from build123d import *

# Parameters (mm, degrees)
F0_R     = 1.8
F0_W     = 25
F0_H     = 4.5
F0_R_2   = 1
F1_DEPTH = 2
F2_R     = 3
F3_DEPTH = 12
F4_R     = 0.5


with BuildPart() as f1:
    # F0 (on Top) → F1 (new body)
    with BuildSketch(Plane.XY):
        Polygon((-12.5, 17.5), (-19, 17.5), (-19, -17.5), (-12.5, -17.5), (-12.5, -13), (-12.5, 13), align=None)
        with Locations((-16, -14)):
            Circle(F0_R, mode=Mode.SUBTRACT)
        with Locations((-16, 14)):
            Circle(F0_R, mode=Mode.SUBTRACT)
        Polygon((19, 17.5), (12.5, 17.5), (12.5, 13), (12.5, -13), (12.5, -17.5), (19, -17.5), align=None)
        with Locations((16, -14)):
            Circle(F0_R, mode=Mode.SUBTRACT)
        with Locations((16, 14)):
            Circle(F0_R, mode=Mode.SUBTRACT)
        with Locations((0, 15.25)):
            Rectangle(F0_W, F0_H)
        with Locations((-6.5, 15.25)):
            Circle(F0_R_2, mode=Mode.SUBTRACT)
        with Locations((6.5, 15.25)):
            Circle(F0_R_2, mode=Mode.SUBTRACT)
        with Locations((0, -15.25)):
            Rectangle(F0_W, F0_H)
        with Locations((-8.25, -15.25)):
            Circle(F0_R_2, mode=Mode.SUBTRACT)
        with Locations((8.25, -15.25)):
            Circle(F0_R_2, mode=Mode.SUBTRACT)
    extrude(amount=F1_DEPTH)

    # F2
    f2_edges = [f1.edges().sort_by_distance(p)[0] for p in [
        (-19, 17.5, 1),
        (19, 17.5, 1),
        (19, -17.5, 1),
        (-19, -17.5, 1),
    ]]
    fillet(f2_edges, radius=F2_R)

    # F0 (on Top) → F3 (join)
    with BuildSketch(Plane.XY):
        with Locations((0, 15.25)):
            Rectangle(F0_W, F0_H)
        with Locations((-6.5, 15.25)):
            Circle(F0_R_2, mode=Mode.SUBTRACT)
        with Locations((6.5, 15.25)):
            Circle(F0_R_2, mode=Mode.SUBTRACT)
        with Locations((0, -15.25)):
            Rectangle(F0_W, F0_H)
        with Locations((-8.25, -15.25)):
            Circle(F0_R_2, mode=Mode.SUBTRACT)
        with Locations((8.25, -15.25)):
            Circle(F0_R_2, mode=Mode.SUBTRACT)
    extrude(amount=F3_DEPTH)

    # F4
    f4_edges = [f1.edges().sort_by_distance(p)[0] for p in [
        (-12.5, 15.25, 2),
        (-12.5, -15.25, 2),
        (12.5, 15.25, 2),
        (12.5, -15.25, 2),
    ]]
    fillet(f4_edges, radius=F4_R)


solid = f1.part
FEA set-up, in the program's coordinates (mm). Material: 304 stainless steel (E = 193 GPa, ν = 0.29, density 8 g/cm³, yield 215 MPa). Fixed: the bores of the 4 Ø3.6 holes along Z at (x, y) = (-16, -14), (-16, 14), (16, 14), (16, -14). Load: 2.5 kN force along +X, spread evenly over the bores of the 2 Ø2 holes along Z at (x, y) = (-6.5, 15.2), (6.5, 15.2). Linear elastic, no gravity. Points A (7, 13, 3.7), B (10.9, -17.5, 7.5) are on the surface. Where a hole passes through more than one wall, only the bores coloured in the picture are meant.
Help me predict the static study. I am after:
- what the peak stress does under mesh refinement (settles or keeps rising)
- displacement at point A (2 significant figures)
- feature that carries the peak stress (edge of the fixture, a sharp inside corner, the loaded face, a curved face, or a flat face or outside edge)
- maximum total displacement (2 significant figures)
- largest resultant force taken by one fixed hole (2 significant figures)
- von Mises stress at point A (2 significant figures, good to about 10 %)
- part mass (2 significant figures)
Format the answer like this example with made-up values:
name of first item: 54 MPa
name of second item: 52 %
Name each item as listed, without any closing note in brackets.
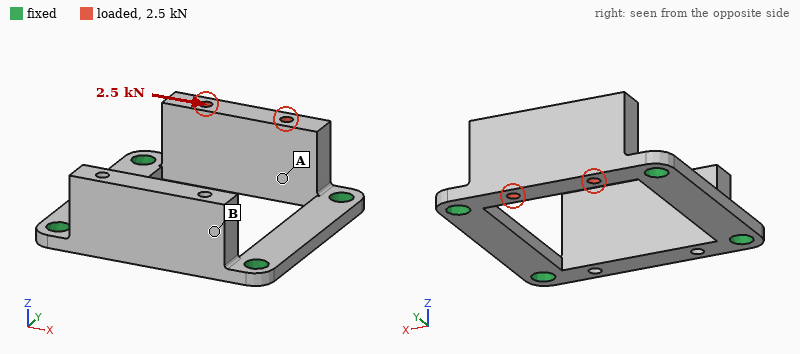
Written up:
what the peak stress does under mesh refinement: keeps rising
displacement at point A: 5.1 µm
feature that carries the peak stress: a sharp inside corner
maximum total displacement: 8.6 µm
largest resultant force taken by one fixed hole: 1.3 kN
von Mises stress at point A: 51 MPa
part mass: 27 g
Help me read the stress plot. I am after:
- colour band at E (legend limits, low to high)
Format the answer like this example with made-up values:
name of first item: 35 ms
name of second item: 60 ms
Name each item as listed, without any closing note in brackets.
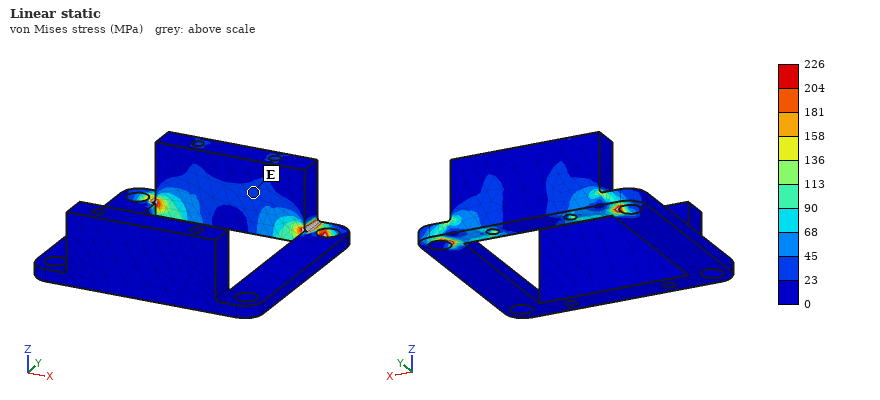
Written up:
colour band at E: 23 to 45 MPa
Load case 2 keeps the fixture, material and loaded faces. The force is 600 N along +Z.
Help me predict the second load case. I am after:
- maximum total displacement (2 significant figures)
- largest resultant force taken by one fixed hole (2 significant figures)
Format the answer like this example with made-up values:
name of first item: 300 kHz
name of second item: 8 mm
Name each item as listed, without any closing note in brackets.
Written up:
maximum total displacement: 7.7 µm
largest resultant force taken by one fixed hole: 360 N
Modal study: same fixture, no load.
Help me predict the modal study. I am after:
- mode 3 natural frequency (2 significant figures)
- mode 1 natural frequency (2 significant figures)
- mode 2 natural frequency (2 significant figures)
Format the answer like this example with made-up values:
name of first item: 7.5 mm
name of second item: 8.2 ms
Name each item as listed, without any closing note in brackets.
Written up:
mode 3 natural frequency: 15 kHz
mode 1 natural frequency: 6300 Hz
mode 2 natural frequency: 6400 Hz
